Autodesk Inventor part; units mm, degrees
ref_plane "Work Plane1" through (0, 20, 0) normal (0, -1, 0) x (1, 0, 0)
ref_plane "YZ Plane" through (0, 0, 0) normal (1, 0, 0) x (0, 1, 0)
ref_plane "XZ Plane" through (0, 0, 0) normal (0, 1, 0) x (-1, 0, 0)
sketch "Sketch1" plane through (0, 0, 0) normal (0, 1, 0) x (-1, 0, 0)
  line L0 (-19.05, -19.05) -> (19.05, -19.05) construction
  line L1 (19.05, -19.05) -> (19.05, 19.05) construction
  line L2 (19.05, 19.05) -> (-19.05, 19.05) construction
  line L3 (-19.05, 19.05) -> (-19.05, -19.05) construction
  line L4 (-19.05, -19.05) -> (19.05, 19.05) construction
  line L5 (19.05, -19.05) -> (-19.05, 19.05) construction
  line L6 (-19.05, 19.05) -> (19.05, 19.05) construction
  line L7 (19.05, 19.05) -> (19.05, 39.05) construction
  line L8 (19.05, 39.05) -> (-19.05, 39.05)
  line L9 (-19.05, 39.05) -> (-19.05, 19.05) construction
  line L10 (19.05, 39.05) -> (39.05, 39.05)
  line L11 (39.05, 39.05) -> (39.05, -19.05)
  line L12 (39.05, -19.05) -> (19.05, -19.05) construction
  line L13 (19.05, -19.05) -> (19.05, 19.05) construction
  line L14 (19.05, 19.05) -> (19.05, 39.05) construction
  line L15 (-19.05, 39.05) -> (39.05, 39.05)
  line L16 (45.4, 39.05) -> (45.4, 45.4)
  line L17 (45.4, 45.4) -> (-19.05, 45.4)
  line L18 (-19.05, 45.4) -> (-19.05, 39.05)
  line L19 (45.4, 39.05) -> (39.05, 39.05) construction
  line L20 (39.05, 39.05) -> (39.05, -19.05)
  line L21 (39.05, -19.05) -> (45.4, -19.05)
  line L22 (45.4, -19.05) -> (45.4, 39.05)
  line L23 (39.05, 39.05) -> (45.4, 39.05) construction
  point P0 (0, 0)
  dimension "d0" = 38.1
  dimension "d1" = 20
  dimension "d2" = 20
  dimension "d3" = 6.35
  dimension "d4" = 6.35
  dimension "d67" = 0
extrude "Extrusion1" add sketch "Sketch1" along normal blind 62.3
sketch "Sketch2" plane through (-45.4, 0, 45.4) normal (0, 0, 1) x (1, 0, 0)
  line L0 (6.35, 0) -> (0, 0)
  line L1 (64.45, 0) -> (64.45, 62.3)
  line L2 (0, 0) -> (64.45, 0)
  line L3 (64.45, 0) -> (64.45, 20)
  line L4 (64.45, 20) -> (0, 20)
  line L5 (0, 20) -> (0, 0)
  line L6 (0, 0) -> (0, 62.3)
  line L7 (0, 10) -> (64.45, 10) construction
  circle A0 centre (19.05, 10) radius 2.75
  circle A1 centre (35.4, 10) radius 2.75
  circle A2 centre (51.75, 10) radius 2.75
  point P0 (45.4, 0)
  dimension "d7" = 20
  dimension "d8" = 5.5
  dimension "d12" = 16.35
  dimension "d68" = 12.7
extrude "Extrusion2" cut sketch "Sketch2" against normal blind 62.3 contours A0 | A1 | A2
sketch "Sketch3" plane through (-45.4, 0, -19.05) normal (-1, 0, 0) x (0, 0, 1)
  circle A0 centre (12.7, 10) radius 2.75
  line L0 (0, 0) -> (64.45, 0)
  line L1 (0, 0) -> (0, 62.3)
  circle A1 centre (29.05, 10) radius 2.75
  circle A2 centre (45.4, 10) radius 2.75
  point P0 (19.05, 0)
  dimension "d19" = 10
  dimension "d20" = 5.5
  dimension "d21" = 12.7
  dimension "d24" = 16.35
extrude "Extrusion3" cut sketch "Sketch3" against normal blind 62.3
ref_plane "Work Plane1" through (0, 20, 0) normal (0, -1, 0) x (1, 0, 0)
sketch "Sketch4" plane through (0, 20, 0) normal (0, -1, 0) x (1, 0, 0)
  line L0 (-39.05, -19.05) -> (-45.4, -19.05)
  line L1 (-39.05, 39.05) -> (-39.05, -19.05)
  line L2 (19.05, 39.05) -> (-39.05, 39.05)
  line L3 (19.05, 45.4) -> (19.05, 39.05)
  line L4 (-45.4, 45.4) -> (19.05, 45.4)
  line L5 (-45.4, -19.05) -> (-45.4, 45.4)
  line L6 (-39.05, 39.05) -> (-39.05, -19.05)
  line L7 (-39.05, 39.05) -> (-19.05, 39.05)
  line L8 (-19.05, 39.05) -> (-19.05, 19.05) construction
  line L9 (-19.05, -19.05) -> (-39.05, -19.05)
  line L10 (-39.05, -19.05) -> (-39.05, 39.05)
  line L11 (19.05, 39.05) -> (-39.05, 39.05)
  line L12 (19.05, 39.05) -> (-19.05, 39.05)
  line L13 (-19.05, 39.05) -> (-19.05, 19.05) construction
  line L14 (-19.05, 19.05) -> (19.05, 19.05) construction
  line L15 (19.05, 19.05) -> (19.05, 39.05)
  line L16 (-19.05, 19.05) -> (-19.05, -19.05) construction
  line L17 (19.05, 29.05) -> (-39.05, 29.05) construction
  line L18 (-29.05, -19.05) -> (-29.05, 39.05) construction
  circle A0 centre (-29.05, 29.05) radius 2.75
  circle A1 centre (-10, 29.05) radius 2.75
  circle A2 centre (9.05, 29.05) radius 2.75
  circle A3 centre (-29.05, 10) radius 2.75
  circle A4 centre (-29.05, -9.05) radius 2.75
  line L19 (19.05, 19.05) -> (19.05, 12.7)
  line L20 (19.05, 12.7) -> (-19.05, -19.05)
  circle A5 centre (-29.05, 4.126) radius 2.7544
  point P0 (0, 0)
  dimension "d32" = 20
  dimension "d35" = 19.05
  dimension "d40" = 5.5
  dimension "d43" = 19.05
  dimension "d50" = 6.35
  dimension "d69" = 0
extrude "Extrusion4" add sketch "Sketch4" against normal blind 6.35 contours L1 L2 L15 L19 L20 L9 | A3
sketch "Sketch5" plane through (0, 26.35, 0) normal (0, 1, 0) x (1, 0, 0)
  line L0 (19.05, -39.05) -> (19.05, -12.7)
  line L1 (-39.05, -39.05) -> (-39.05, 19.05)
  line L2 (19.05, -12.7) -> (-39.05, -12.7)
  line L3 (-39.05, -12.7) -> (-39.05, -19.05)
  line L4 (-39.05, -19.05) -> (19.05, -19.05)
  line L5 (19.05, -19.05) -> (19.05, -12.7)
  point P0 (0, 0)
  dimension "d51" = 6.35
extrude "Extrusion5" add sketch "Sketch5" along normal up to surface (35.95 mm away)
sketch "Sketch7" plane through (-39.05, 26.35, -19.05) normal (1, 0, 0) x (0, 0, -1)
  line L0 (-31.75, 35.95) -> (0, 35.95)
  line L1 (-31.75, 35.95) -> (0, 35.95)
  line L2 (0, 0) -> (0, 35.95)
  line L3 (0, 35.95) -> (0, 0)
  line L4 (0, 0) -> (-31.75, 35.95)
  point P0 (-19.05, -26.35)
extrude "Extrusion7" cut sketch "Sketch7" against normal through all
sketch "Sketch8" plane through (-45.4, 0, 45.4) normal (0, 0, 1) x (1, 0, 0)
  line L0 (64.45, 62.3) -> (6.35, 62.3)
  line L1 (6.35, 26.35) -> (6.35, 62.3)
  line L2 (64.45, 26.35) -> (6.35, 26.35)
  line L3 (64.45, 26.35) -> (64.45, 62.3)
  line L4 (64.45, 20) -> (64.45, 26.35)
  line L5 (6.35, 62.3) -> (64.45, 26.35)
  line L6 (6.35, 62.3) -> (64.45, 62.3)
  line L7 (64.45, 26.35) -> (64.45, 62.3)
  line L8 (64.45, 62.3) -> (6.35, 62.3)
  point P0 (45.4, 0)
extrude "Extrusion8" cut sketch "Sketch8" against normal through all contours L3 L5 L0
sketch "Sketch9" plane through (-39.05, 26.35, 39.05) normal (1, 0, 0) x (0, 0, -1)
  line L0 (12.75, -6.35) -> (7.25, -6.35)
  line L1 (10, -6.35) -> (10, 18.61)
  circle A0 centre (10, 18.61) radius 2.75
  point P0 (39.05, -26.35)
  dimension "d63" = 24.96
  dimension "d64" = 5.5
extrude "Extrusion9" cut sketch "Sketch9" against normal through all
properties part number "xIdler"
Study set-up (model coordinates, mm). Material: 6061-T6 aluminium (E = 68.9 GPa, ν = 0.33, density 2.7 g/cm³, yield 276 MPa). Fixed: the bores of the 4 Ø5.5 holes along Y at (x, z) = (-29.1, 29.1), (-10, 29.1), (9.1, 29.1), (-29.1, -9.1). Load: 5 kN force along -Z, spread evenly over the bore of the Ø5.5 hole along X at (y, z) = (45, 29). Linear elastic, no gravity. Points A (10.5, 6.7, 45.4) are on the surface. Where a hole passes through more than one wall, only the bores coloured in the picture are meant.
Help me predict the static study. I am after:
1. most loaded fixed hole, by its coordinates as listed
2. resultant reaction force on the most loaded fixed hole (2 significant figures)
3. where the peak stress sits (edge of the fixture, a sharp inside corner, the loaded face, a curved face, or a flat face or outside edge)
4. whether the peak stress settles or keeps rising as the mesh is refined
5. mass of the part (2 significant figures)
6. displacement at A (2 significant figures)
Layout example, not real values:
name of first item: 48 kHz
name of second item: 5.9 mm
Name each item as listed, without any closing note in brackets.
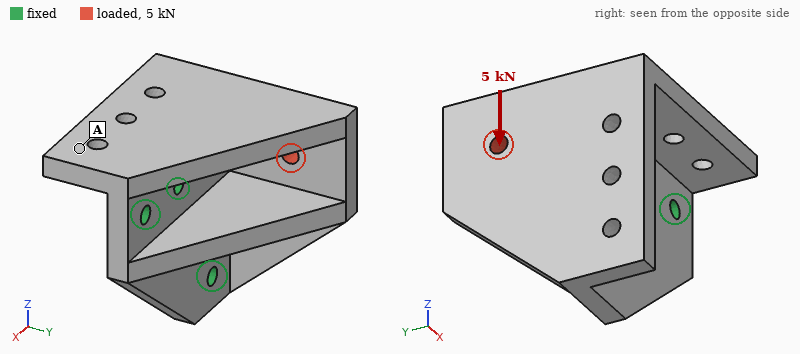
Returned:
most loaded fixed hole, by its coordinates as listed: (-29.1, 29.1)
resultant reaction force on the most loaded fixed hole: 4.0 kN
where the peak stress sits: edge of the fixture
whether the peak stress settles or keeps rising as the mesh is refined: keeps rising
mass of the part: 160 g
displacement at A: 14 µm
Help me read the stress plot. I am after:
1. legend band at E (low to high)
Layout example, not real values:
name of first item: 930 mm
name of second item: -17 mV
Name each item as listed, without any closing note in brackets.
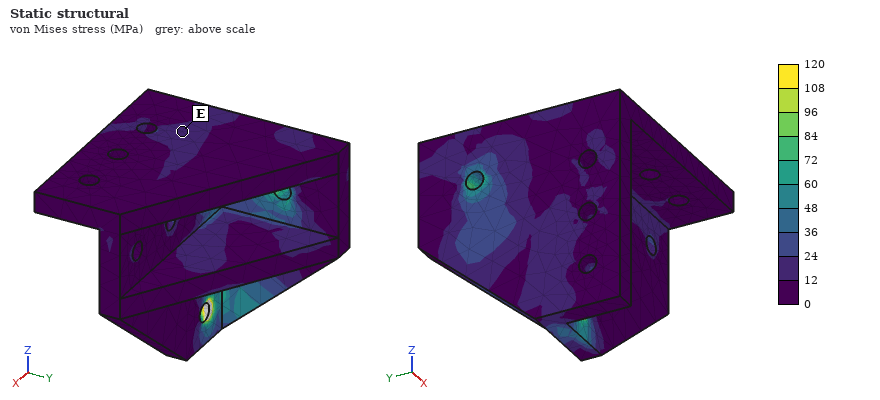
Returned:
legend band at E: 12 to 24 MPa
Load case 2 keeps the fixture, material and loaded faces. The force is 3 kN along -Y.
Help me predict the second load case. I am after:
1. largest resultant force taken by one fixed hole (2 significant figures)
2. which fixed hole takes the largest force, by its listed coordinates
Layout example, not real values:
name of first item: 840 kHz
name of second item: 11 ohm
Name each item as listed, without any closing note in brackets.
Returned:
largest resultant force taken by one fixed hole: 3.3 kN
which fixed hole takes the largest force, by its listed coordinates: (-29.1, 29.1)
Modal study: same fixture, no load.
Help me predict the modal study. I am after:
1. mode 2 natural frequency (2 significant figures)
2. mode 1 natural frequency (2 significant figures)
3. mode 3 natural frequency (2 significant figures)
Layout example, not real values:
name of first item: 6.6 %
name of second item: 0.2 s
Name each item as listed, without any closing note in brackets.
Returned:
mode 2 natural frequency: 6000 Hz
mode 1 natural frequency: 5500 Hz
mode 3 natural frequency: 7000 Hz
